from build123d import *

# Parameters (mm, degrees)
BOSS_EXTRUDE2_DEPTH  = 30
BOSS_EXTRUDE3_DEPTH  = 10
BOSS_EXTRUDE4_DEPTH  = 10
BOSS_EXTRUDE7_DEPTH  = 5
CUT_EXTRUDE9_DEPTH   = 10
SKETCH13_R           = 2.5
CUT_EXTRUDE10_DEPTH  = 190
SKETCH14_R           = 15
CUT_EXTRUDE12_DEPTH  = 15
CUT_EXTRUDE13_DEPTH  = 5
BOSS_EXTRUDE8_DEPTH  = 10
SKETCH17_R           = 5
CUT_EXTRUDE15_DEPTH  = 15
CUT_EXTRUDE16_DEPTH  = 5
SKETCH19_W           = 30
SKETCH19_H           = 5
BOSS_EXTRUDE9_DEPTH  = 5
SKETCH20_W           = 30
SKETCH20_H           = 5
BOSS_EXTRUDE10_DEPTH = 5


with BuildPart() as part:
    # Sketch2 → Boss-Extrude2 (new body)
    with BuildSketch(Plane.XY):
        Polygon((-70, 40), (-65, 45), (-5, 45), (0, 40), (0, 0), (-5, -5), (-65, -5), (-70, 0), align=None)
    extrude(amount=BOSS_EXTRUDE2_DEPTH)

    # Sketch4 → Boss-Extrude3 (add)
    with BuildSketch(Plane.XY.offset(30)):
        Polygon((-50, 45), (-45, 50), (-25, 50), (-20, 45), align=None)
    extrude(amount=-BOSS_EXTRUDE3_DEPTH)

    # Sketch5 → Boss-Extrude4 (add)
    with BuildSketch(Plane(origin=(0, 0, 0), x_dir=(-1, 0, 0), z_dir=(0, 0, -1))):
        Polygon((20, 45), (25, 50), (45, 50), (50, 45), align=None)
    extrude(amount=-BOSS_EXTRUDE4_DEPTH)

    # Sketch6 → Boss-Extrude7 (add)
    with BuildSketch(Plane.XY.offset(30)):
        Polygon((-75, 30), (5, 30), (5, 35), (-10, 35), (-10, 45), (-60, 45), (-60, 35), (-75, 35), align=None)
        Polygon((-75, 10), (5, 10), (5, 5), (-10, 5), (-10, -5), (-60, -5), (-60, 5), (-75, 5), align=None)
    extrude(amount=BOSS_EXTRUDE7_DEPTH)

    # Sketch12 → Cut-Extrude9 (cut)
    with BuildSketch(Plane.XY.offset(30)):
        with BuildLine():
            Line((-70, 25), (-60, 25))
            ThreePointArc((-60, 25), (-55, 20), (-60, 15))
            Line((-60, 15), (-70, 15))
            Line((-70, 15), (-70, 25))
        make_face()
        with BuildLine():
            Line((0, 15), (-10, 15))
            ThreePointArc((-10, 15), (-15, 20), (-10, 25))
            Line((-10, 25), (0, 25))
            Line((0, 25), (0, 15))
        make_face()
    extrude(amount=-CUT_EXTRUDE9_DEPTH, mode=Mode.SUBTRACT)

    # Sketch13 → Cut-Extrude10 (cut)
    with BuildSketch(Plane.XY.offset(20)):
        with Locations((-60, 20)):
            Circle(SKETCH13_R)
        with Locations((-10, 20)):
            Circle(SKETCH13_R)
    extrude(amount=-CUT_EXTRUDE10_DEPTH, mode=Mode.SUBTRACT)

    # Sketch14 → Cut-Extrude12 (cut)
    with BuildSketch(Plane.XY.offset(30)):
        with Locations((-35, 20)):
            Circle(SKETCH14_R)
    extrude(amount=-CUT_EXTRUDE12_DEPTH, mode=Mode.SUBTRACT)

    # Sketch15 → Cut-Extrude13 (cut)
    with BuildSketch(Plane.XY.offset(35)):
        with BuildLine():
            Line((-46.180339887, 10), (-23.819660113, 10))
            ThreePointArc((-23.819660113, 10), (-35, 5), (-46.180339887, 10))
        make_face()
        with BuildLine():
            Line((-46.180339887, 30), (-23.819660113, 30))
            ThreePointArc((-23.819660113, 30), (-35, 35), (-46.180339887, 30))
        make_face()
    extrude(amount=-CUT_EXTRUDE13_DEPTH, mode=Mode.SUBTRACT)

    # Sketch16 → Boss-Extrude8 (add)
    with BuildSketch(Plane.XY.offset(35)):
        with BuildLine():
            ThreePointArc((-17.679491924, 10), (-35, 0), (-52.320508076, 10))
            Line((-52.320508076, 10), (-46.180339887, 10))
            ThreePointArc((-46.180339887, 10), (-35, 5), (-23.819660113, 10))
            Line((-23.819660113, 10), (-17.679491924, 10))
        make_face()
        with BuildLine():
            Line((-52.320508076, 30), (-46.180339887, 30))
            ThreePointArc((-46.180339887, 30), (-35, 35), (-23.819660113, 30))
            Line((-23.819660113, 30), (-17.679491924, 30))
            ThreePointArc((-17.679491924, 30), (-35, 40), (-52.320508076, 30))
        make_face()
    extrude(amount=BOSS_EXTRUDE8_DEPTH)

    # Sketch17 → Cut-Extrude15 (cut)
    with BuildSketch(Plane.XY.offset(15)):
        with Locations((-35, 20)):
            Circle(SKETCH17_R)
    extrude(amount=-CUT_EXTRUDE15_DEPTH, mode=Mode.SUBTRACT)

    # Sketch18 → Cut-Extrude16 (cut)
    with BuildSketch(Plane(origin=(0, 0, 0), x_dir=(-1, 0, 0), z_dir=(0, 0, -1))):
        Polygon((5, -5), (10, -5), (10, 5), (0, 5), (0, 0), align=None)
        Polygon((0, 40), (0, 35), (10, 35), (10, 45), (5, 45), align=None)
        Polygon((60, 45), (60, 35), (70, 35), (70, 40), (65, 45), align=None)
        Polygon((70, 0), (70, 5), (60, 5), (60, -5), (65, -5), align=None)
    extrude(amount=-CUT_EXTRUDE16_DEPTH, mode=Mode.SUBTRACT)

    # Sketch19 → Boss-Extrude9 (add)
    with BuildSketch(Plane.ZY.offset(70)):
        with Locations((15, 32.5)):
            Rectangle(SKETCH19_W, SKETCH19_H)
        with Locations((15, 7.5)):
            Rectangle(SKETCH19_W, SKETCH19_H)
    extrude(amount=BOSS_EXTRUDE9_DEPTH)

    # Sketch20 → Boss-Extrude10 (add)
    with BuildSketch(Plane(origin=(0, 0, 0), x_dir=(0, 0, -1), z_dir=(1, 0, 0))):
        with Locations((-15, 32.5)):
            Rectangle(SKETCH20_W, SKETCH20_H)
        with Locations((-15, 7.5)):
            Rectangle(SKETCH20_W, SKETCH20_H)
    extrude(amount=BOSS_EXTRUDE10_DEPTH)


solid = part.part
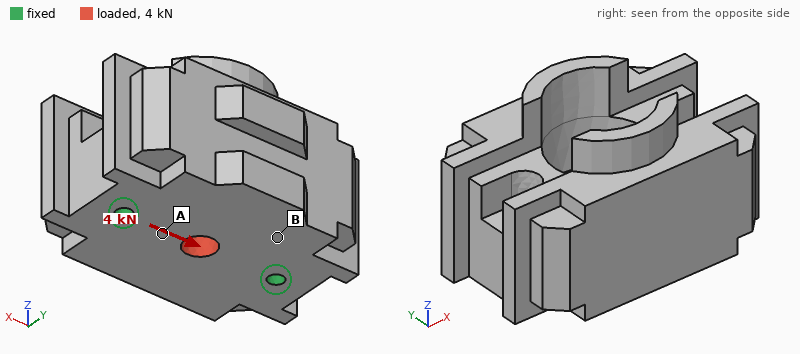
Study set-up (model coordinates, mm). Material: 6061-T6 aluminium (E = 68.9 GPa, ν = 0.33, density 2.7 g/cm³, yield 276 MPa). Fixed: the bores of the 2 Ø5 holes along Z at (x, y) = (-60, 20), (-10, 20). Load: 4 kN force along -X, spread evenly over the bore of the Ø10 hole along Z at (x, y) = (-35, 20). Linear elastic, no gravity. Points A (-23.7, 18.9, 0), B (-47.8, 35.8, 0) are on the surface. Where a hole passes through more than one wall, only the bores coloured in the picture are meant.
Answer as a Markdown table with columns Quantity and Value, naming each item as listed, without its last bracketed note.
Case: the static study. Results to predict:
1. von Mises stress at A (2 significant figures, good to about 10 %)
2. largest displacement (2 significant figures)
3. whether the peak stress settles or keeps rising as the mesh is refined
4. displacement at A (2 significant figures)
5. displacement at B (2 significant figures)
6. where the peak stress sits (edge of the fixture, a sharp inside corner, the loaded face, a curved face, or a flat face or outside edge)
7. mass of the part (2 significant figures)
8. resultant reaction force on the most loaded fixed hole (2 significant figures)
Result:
| Quantity | Value |
|---|---|
| von Mises stress at A | 8.4 MPa |
| largest displacement | 2.3 µm |
| whether the peak stress settles or keeps rising as the mesh is refined | keeps rising |
| displacement at A | 1.5 µm |
| displacement at B | 1.2 µm |
| where the peak stress sits | edge of the fixture |
| mass of the part | 280 g |
| resultant reaction force on the most loaded fixed hole | 2.0 kN |
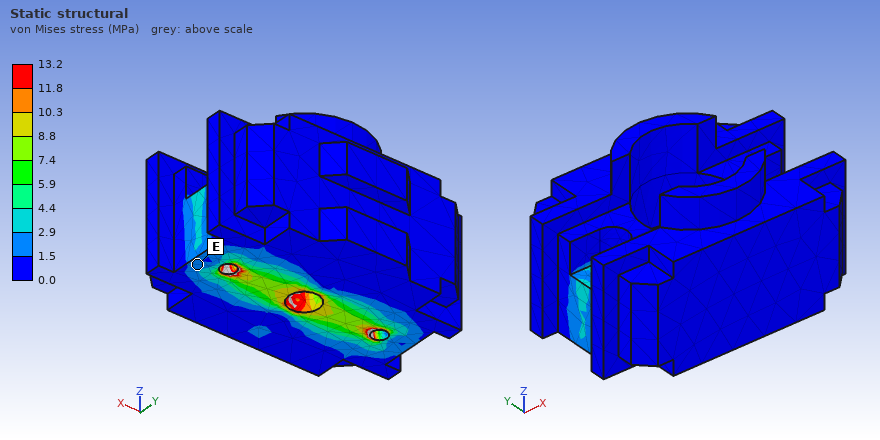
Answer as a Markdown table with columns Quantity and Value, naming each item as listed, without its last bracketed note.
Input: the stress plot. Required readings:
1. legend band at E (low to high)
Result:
| Quantity | Value |
|---|---|
| legend band at E | 1.5 to 2.9 MPa |
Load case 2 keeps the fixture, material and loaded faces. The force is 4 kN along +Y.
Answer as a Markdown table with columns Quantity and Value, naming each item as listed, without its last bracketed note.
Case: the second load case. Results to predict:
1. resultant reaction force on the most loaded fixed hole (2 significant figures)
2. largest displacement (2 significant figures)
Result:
| Quantity | Value |
|---|---|
| resultant reaction force on the most loaded fixed hole | 2.0 kN |
| largest displacement | 4.0 µm |
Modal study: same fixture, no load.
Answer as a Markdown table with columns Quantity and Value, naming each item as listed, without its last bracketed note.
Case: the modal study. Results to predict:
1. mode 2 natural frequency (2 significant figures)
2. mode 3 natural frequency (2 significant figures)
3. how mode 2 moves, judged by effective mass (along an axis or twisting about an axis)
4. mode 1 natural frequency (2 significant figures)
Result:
| Quantity | Value |
|---|---|
| mode 2 natural frequency | 12 kHz |
| mode 3 natural frequency | 14 kHz |
| how mode 2 moves, judged by effective mass | along Z |
| mode 1 natural frequency | 7700 Hz |
